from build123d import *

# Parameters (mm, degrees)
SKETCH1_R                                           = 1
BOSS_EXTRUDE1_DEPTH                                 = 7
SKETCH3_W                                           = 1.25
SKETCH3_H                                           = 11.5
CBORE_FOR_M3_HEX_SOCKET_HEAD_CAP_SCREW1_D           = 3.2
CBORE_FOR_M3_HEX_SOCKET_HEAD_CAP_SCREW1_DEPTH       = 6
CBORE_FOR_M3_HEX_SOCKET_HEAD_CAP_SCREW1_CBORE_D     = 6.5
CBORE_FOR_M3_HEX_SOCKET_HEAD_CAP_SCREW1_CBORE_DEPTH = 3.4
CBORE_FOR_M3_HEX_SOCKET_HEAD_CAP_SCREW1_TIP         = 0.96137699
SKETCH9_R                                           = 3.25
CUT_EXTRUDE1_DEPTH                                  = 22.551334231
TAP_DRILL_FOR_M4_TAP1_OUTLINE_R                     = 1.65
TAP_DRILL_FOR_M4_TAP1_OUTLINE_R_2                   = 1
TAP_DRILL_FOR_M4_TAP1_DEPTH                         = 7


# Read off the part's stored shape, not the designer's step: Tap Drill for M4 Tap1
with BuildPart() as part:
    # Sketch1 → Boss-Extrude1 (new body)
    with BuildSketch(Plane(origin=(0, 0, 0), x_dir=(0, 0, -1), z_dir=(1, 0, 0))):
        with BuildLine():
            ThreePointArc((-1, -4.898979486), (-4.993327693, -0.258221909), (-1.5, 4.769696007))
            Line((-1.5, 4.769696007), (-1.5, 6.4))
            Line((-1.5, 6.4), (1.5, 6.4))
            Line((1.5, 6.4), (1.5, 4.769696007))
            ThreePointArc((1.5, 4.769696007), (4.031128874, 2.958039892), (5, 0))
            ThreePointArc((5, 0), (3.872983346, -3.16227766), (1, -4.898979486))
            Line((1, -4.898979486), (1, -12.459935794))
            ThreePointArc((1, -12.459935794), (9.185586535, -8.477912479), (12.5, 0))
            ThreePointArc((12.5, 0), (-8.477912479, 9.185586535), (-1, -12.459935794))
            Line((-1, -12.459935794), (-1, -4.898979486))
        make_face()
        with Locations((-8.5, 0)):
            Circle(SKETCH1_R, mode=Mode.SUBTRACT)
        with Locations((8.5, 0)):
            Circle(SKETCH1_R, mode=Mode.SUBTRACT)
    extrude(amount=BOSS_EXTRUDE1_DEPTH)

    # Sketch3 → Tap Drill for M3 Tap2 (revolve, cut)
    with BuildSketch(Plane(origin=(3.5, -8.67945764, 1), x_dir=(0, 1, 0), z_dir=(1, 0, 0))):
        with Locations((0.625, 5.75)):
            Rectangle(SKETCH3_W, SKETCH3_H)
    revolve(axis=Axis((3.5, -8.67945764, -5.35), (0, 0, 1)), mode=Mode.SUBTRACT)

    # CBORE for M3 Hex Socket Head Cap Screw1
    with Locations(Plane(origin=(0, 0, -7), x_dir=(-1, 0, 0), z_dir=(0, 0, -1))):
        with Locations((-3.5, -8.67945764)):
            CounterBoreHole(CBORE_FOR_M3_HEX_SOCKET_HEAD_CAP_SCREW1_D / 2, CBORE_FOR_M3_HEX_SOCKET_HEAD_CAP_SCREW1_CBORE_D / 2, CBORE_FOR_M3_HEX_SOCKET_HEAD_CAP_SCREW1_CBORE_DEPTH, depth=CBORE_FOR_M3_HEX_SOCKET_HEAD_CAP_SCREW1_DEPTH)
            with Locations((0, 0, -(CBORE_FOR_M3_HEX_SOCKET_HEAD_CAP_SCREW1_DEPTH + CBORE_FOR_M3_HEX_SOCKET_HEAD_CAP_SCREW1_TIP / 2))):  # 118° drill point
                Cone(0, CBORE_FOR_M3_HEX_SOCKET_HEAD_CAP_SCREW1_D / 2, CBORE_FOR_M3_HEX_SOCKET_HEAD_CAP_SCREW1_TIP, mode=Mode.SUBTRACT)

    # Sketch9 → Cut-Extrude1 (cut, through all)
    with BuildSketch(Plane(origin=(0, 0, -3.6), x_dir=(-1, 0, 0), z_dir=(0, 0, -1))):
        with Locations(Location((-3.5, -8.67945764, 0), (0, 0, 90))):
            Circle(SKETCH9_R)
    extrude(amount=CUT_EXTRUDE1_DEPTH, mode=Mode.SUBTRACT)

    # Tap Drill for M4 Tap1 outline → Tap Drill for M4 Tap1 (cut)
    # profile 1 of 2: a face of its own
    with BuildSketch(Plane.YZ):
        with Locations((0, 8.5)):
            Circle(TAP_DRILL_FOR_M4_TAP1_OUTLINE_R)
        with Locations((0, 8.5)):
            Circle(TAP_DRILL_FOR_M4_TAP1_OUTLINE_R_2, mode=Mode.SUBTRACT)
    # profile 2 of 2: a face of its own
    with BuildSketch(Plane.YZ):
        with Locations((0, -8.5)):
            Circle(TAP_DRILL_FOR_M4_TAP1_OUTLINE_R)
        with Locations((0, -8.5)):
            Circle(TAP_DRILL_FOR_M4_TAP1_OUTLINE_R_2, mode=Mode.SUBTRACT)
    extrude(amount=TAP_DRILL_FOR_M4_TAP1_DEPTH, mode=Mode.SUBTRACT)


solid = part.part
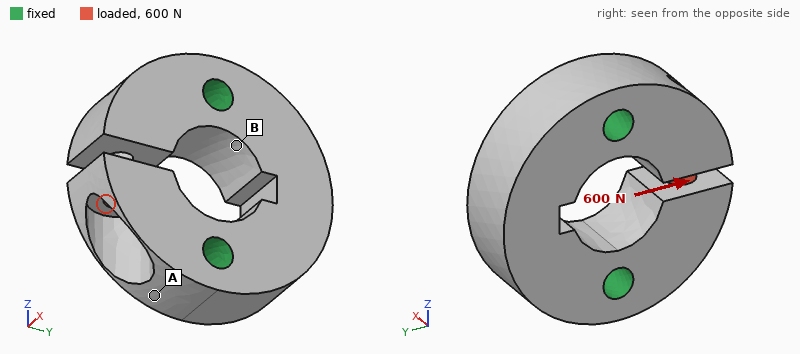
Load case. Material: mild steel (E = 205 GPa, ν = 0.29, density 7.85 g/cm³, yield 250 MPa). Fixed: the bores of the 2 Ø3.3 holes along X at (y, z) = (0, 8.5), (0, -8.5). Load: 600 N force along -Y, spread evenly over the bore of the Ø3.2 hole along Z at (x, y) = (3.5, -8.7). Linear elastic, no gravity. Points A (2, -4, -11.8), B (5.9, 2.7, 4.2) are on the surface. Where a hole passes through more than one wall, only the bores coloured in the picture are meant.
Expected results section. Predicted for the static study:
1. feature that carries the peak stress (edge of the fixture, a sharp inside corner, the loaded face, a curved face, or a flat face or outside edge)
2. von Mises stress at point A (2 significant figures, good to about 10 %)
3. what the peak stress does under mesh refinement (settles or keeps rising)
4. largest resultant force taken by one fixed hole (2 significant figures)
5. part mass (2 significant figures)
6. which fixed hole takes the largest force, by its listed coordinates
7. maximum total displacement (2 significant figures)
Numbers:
a sharp inside corner
22 MPa
keeps rising
570 N
19 g
(0, -8.5)
11 µm
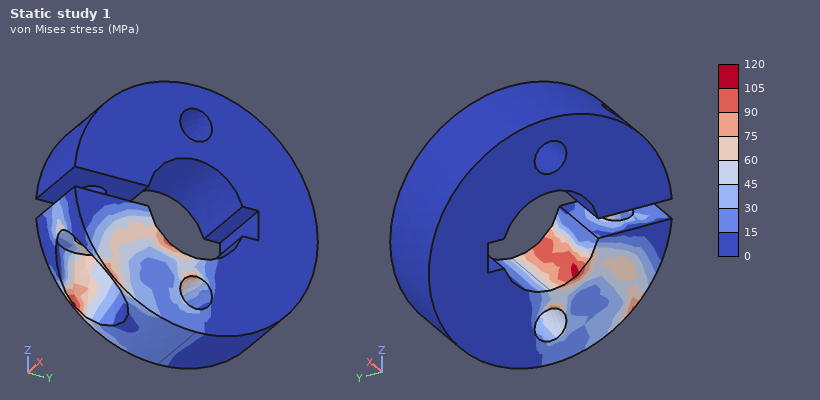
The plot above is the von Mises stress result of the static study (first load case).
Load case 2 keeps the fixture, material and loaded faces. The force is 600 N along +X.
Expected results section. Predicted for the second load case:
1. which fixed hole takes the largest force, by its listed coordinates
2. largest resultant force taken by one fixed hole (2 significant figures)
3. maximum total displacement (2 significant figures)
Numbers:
(0, -8.5)
600 N
20 µm
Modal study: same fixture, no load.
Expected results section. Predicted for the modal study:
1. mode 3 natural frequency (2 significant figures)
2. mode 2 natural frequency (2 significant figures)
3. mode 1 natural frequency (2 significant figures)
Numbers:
31 kHz
31 kHz
29 kHz
